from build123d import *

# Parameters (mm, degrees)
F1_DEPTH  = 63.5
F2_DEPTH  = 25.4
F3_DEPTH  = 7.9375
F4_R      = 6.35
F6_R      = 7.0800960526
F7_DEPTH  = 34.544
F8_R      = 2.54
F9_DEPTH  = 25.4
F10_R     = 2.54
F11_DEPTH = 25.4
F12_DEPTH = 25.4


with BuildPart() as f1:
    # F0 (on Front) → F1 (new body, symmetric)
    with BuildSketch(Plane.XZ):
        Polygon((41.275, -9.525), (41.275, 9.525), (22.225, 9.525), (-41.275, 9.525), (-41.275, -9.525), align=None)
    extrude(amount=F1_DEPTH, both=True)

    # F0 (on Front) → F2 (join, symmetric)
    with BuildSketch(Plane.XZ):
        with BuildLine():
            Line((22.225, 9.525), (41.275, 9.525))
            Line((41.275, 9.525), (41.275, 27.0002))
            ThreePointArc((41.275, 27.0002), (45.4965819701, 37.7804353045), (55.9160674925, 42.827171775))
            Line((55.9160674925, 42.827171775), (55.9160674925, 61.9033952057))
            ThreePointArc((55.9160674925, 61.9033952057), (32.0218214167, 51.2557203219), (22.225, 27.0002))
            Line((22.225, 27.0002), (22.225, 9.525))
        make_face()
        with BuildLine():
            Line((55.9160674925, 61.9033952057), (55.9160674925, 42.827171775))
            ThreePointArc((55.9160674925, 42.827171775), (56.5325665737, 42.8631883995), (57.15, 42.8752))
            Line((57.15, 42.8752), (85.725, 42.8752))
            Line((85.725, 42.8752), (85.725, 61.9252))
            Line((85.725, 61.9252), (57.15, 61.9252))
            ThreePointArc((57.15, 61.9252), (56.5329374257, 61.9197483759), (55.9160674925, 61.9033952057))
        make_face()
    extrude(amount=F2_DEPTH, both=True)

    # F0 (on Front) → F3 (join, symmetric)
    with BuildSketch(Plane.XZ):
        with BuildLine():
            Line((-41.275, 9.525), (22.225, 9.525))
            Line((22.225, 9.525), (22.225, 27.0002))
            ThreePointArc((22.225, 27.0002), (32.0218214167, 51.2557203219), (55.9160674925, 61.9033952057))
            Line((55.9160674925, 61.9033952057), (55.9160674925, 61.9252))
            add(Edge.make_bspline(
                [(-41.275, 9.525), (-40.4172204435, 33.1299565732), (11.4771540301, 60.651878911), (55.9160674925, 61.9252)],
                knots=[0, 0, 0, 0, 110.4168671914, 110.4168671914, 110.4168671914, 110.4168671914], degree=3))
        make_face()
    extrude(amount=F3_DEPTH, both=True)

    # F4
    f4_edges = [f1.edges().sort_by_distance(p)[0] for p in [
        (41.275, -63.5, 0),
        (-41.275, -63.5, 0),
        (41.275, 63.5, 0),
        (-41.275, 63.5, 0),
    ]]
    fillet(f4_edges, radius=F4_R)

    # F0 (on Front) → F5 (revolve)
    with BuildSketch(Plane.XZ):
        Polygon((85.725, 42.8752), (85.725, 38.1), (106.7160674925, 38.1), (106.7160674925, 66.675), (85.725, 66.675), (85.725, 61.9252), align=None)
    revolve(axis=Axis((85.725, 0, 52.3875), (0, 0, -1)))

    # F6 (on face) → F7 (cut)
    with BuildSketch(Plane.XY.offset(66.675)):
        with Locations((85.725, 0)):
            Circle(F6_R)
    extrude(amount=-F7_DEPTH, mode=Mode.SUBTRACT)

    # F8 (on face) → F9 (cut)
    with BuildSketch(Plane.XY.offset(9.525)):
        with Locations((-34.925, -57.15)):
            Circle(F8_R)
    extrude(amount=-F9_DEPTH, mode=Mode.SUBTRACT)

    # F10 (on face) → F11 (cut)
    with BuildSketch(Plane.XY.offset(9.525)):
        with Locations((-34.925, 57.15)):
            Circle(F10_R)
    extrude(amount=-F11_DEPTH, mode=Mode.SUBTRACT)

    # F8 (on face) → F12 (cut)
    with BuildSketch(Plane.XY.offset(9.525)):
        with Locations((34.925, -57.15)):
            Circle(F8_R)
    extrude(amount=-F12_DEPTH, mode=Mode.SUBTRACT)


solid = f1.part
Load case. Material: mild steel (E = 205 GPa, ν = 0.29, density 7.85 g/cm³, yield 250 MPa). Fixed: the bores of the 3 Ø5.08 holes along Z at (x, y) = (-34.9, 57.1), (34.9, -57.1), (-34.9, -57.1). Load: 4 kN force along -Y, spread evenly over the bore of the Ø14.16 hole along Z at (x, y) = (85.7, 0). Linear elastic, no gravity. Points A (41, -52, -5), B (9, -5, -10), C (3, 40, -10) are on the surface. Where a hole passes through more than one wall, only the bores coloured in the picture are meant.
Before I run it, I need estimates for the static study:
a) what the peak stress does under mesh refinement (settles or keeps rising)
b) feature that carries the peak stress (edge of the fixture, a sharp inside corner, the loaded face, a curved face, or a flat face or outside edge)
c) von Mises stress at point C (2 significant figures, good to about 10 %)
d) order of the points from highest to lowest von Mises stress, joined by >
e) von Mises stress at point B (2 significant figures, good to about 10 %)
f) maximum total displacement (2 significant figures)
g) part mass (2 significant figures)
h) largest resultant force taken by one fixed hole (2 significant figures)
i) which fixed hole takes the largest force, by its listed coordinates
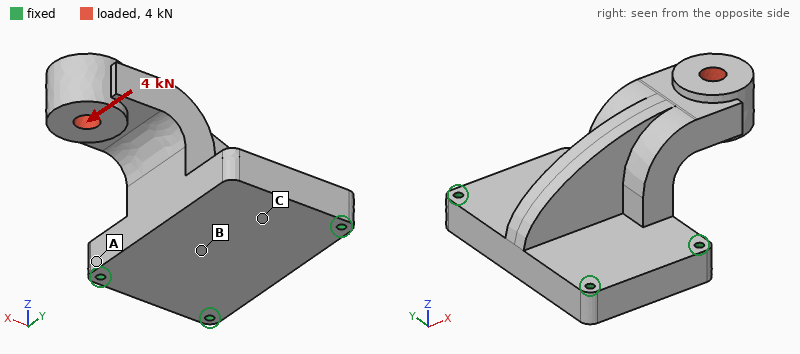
keeps rising
edge of the fixture
9.4 MPa
B > C > A
17 MPa
90 µm
2.7 kg
3.4 kN
(-34.9, 57.1)
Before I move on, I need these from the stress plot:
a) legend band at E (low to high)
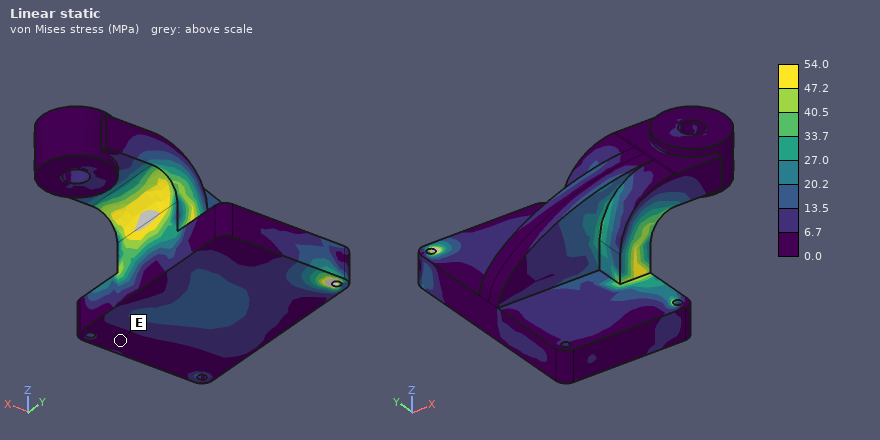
0.0 to 6.7 MPa
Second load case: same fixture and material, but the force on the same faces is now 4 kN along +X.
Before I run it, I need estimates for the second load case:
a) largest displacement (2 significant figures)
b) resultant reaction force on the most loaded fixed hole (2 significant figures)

61 µm
3.0 kN
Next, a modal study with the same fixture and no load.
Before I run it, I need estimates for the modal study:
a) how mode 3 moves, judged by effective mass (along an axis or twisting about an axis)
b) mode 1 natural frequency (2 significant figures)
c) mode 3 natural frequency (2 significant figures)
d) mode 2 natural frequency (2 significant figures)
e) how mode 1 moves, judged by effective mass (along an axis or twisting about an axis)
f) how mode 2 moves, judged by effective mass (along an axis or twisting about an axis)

along Z
1200 Hz
3300 Hz
2100 Hz
along Z
along Y
